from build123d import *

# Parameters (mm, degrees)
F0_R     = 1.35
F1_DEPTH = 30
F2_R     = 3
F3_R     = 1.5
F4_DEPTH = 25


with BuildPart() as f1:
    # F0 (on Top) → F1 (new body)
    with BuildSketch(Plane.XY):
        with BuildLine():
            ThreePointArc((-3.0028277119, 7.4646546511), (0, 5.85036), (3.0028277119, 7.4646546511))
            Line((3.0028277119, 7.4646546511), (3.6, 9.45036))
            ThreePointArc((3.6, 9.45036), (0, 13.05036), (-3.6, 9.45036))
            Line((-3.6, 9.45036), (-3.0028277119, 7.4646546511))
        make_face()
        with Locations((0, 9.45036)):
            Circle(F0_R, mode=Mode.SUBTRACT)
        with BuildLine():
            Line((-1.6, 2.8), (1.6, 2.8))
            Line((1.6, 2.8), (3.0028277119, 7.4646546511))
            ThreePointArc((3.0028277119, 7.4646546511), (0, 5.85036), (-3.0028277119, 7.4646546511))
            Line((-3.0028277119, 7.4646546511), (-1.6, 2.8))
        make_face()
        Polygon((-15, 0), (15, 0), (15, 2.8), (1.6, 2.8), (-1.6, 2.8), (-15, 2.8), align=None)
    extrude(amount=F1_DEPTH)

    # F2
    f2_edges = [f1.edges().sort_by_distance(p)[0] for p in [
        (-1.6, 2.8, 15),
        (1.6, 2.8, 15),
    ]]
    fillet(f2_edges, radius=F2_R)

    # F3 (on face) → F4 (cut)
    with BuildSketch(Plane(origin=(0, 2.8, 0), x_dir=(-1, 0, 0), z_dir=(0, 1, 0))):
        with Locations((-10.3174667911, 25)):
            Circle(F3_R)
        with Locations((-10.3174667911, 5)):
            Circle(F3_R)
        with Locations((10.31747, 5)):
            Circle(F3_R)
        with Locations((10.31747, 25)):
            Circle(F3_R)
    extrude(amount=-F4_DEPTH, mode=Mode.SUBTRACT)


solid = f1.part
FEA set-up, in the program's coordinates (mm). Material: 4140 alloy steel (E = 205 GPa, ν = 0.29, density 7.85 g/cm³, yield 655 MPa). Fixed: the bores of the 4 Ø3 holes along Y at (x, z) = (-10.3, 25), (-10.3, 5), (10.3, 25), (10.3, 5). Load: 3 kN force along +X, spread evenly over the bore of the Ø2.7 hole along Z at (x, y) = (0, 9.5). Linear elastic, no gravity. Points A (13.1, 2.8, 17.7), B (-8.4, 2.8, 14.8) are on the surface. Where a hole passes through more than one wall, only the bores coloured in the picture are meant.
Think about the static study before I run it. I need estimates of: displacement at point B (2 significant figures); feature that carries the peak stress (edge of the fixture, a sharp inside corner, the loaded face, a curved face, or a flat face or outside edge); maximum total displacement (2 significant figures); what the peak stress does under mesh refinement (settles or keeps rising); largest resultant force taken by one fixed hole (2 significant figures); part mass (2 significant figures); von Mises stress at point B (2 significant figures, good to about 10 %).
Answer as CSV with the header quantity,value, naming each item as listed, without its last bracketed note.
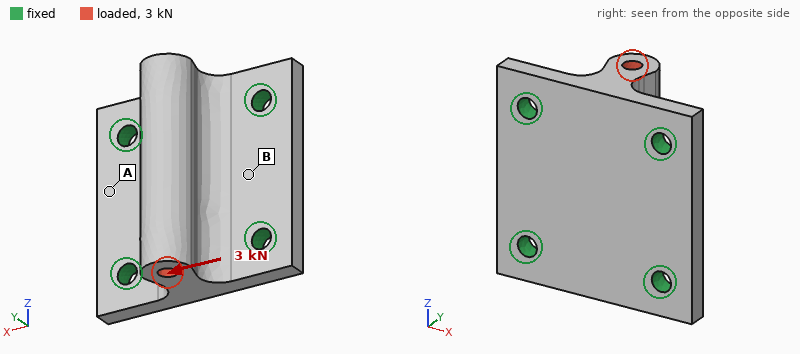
quantity,value
displacement at point B,4.2 µm
feature that carries the peak stress,edge of the fixture
maximum total displacement,20 µm
what the peak stress does under mesh refinement,keeps rising
largest resultant force taken by one fixed hole,1.1 kN
part mass,33 g
von Mises stress at point B,41 MPa
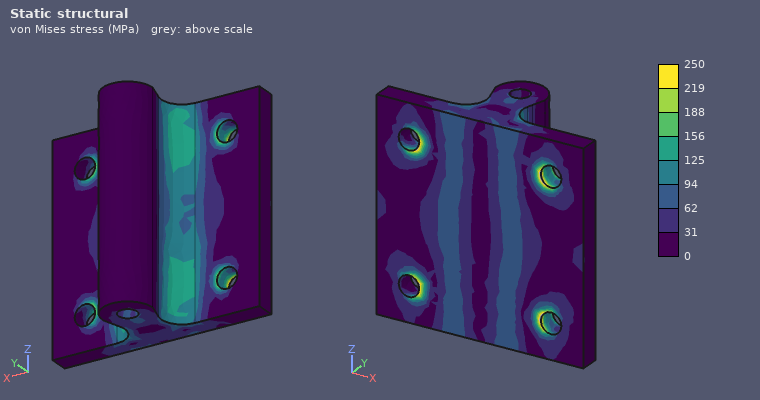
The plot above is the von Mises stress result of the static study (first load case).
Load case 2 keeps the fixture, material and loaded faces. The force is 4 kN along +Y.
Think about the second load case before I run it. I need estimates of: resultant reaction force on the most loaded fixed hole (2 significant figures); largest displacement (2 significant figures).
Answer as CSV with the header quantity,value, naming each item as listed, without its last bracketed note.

quantity,value
resultant reaction force on the most loaded fixed hole,1.1 kN
largest displacement,12 µm
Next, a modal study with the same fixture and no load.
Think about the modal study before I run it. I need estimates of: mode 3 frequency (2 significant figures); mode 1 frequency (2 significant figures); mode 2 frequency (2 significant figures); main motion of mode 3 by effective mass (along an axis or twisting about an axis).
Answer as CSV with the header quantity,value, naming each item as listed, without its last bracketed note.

quantity,value
mode 3 frequency,23 kHz
mode 1 frequency,21 kHz
mode 2 frequency,21 kHz
main motion of mode 3 by effective mass,along X
